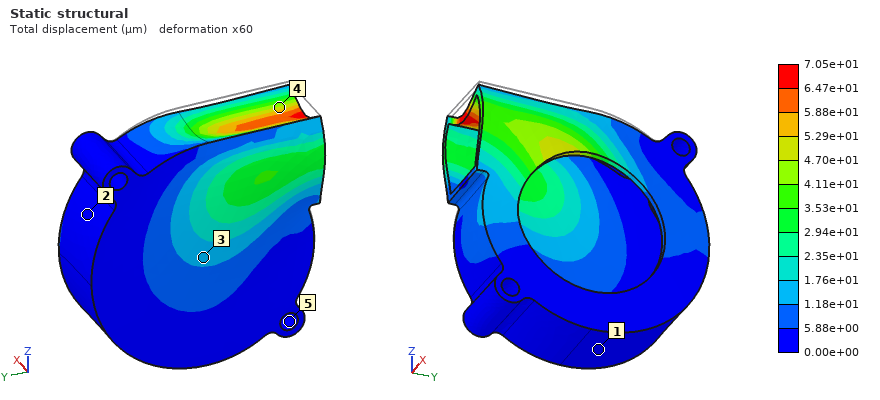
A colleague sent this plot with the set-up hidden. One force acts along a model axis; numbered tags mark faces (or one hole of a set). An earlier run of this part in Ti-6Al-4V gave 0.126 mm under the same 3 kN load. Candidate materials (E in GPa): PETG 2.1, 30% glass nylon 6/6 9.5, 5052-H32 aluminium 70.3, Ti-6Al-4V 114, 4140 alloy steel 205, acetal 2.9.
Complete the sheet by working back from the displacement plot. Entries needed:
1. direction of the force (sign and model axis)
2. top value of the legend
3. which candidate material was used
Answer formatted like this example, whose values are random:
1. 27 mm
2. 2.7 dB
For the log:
1. -Z
2. 7.05e+01 µm
3. 4140 alloy steel
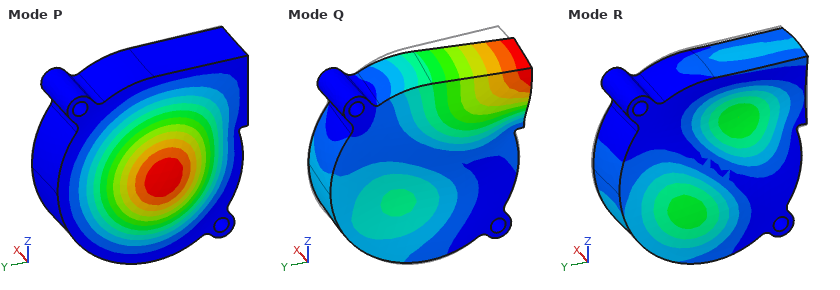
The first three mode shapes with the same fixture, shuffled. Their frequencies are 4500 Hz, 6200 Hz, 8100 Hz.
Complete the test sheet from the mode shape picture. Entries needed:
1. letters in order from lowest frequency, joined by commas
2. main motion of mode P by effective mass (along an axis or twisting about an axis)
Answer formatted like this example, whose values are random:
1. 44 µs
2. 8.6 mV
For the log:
1. P, Q, R
2. along X
